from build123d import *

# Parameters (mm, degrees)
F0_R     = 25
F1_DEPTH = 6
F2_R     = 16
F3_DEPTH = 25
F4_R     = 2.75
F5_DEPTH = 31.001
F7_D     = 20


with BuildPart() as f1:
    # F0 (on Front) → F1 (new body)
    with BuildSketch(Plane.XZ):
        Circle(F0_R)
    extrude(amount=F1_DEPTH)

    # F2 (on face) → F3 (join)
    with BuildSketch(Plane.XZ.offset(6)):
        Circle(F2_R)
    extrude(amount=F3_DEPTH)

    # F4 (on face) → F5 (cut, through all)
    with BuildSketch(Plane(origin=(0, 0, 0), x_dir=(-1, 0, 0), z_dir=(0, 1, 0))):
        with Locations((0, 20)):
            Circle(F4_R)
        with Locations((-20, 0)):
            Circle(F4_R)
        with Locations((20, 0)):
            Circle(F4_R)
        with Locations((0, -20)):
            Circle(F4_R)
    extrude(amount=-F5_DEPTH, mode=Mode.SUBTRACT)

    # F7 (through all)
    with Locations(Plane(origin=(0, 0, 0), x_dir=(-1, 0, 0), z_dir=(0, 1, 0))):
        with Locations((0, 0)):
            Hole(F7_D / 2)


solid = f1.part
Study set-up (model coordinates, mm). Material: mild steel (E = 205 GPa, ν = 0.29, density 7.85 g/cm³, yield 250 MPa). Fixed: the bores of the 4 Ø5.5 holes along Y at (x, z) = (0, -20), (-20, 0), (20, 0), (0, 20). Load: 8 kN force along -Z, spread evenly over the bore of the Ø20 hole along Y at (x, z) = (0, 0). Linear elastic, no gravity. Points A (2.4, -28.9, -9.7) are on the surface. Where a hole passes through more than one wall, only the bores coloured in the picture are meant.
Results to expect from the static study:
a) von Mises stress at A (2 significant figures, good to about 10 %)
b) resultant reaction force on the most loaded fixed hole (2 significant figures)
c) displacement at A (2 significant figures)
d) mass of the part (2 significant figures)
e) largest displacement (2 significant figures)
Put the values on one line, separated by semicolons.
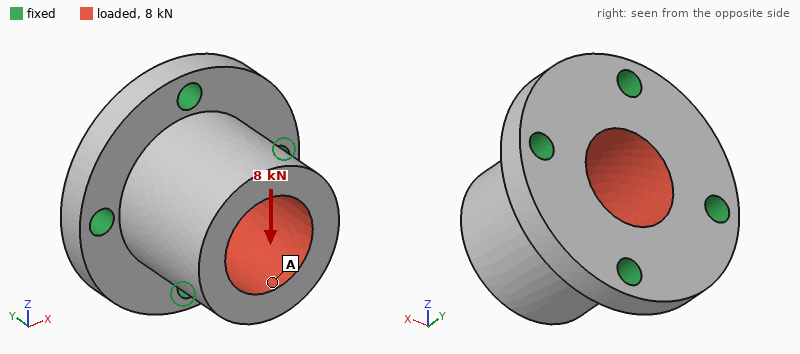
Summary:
12 MPa; 3.5 kN; 10 µm; 170 g; 11 µm
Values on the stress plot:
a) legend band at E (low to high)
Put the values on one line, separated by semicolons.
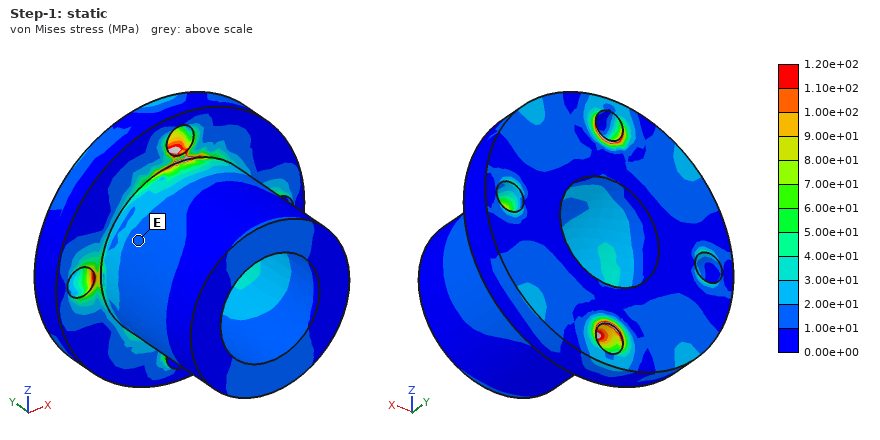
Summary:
1.00e+01 to 2.00e+01 MPa
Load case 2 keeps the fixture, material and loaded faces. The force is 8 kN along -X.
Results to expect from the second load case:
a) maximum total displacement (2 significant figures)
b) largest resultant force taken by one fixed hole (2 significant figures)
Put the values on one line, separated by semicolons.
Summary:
11 µm; 3.5 kN
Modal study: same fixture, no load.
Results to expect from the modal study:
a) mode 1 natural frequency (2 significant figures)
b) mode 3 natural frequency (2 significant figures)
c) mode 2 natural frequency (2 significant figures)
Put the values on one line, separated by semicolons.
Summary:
14 kHz; 23 kHz; 14 kHz
